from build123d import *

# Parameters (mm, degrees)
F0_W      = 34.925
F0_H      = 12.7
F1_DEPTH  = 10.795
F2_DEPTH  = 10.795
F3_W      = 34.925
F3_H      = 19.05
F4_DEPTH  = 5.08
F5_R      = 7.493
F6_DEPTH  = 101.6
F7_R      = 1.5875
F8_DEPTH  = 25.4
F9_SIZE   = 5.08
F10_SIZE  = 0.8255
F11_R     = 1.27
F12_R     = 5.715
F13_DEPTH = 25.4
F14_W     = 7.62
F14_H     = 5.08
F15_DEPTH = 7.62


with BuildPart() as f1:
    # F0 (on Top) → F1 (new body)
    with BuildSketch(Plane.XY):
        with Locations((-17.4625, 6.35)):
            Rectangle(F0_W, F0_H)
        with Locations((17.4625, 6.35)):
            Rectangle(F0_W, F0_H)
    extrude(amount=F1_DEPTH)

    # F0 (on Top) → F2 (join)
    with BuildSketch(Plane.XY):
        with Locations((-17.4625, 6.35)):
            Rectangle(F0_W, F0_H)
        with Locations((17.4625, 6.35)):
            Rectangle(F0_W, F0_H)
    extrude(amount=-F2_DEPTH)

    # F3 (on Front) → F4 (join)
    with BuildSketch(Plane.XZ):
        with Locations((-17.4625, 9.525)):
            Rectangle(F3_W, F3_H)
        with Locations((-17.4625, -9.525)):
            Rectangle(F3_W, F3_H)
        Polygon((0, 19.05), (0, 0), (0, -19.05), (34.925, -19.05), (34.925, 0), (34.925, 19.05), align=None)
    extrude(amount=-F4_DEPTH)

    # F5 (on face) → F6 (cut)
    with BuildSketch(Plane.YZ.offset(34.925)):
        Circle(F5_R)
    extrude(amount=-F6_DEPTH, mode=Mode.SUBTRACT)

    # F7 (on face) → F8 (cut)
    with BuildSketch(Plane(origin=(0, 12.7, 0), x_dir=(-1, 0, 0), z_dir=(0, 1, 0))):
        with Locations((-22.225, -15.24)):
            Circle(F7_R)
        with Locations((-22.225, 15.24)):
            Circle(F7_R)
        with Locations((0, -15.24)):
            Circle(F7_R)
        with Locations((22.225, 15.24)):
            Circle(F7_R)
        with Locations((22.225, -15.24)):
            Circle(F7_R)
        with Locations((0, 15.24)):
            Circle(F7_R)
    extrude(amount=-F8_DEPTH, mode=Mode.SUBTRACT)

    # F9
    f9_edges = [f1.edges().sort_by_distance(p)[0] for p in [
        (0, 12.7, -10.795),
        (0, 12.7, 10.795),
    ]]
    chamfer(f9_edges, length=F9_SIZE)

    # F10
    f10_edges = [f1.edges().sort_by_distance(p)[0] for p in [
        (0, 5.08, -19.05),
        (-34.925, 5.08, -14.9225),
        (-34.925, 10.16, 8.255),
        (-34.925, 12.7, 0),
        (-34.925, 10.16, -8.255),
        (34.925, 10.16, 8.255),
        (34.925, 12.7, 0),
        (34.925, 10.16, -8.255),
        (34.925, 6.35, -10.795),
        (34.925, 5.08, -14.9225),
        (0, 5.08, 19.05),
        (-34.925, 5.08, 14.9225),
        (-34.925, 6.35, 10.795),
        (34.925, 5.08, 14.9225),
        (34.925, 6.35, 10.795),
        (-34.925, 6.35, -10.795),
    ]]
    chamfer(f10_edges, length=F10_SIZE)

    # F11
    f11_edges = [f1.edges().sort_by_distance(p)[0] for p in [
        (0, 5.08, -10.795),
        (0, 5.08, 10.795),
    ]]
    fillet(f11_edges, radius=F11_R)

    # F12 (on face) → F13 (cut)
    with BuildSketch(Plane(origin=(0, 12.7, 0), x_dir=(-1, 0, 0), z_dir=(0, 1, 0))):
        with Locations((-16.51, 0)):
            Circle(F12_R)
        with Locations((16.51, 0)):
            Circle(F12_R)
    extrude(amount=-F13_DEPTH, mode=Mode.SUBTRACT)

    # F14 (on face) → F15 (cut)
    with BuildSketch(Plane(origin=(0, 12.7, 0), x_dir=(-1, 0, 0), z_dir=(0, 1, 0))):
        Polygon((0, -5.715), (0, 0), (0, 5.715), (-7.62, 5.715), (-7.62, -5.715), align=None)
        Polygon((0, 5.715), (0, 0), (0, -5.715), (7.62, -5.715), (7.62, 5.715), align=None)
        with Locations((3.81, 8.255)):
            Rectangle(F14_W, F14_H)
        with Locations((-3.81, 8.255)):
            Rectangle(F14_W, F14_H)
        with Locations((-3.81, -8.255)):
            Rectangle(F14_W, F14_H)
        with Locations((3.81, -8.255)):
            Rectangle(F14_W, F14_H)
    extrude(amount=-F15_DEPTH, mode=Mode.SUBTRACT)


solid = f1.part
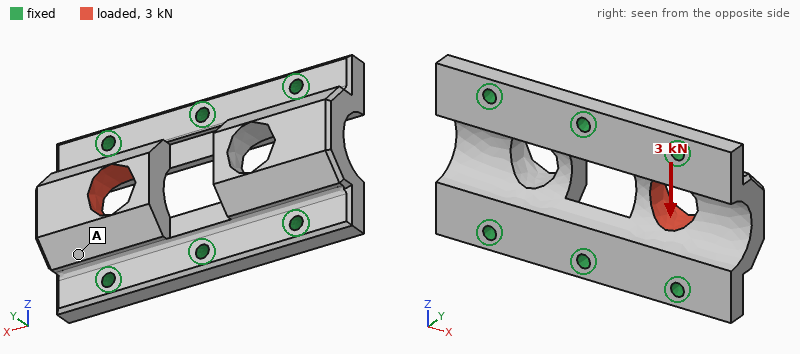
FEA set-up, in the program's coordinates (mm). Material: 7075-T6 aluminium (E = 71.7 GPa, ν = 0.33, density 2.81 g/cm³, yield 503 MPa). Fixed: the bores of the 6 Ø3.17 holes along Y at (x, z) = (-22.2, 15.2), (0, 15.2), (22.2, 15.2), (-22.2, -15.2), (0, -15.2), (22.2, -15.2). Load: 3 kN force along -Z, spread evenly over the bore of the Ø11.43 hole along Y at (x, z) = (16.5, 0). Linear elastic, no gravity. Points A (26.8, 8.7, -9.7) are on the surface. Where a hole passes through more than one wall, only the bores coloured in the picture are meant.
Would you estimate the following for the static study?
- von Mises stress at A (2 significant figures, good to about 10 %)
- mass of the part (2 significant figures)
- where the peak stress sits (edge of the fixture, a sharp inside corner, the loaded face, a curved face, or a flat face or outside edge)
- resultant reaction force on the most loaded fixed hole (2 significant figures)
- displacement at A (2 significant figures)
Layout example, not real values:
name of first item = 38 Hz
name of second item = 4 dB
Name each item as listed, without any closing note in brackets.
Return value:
von Mises stress at A = 9.3 MPa
mass of the part = 39 g
where the peak stress sits = a curved face
resultant reaction force on the most loaded fixed hole = 1.3 kN
displacement at A = 4.8 µm
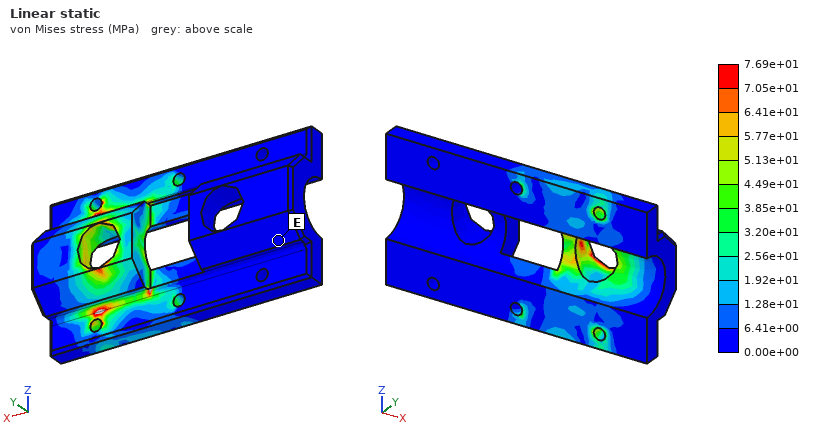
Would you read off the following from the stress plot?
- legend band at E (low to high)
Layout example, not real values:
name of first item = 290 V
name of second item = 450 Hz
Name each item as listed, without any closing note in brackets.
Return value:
legend band at E = 0.00e+00 to 6.41e+00 MPa
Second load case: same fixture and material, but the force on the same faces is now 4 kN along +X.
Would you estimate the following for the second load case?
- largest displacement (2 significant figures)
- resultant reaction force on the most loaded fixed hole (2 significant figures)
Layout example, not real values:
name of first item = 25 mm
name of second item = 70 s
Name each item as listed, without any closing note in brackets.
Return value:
largest displacement = 32 µm
resultant reaction force on the most loaded fixed hole = 1.3 kN
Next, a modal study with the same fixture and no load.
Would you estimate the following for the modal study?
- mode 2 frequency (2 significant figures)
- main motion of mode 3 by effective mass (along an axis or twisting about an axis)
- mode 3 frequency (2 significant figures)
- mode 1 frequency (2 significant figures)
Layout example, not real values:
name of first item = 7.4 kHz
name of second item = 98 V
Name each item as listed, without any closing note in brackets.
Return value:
mode 2 frequency = 17 kHz
main motion of mode 3 by effective mass = along Y
mode 3 frequency = 27 kHz
mode 1 frequency = 17 kHz
